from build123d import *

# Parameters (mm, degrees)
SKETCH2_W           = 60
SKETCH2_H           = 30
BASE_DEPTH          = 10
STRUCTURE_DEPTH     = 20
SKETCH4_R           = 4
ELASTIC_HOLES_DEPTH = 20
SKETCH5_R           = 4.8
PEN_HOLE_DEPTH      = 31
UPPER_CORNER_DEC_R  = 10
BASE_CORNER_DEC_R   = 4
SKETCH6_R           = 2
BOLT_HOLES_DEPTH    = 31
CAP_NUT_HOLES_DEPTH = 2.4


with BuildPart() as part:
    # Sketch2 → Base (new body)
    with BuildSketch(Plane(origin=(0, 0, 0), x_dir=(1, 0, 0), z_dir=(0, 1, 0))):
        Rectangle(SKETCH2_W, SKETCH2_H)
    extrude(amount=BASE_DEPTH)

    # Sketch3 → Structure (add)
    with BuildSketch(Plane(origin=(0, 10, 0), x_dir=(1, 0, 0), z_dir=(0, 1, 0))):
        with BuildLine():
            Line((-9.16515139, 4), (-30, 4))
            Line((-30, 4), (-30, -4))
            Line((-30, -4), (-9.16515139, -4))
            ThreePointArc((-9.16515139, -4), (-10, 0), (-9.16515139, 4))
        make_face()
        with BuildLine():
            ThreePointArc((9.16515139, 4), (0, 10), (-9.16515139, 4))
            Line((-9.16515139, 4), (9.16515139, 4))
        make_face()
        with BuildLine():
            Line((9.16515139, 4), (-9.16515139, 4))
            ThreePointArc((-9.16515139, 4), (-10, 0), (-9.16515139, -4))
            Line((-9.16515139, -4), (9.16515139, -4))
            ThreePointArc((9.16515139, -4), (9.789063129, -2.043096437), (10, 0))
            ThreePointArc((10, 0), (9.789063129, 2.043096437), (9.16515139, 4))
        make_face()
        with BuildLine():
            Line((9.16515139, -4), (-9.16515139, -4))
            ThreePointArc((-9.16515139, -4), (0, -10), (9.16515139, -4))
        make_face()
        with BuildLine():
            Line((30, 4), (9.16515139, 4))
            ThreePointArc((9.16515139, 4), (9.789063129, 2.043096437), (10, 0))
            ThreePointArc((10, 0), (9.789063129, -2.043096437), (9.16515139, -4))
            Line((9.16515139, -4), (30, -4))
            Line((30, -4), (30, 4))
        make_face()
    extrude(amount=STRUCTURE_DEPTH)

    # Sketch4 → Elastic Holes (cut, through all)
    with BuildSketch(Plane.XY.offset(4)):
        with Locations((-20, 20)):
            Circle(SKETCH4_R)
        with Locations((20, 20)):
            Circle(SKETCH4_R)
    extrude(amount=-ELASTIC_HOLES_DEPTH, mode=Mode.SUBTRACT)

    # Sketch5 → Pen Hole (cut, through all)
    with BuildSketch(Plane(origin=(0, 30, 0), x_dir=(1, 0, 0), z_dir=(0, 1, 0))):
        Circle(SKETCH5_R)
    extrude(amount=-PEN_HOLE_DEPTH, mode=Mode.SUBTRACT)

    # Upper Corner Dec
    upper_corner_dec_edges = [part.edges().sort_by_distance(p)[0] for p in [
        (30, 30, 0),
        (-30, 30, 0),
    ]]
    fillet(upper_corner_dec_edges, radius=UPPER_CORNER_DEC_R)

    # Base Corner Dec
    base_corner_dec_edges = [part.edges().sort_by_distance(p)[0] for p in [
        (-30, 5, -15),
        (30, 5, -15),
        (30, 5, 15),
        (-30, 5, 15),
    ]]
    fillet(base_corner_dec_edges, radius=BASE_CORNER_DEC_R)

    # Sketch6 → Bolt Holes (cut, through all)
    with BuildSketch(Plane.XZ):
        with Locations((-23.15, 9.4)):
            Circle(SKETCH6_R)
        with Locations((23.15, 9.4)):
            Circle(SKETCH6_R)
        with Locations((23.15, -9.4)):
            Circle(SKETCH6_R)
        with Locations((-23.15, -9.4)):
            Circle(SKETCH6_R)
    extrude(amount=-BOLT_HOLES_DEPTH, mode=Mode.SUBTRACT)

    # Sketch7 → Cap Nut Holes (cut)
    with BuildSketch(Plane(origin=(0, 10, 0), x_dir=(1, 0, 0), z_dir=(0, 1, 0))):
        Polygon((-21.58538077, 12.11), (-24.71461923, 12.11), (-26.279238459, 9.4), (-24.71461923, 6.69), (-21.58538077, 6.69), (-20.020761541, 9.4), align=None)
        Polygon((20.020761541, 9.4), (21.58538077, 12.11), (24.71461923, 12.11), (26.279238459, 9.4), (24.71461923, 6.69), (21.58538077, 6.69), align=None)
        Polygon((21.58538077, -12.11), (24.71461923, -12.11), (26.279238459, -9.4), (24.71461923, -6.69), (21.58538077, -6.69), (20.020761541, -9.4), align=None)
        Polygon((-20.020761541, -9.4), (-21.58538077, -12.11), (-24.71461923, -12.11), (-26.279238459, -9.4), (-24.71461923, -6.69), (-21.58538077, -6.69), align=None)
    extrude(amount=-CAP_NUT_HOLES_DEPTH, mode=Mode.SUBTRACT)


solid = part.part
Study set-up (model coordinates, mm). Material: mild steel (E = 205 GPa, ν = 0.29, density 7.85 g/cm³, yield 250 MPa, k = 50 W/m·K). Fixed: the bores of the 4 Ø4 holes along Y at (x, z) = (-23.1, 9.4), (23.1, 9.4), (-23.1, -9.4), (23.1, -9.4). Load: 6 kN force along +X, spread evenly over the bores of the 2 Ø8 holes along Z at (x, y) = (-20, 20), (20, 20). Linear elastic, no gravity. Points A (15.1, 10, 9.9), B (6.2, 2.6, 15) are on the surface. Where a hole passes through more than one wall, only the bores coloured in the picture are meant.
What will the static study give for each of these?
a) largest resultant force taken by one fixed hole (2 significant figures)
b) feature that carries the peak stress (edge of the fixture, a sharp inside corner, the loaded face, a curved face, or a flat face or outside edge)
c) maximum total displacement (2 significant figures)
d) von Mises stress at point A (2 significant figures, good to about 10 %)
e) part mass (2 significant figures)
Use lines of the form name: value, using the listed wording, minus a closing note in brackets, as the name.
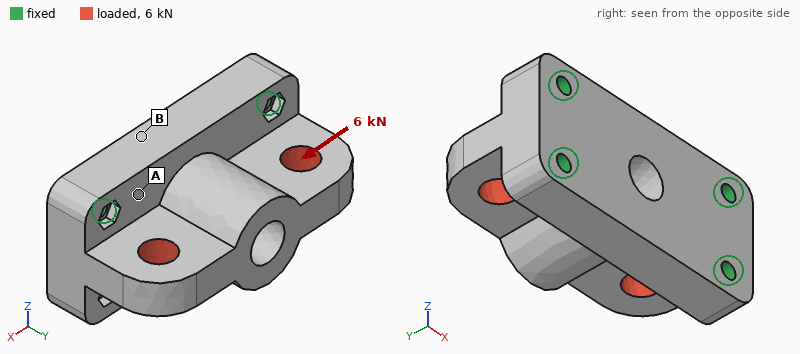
largest resultant force taken by one fixed hole: 1.8 kN
feature that carries the peak stress: edge of the fixture
maximum total displacement: 5.3 µm
von Mises stress at point A: 10 MPa
part mass: 210 g
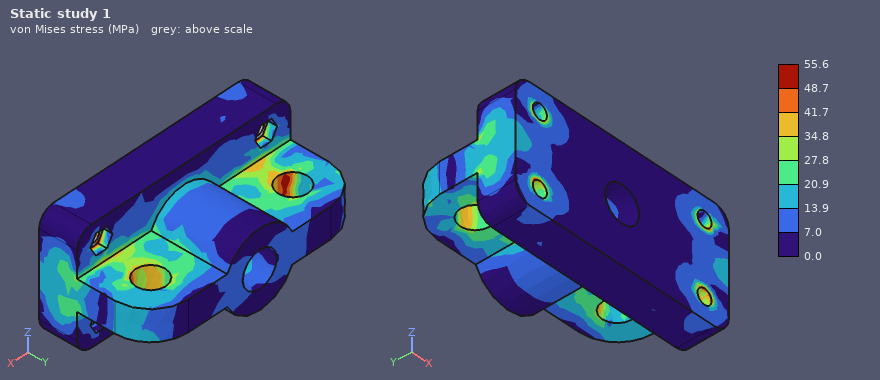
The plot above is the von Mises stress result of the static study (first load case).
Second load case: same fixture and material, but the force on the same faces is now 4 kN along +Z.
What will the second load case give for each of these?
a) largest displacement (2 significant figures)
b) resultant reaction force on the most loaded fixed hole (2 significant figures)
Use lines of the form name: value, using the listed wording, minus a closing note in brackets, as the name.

largest displacement: 13 µm
resultant reaction force on the most loaded fixed hole: 1.9 kN
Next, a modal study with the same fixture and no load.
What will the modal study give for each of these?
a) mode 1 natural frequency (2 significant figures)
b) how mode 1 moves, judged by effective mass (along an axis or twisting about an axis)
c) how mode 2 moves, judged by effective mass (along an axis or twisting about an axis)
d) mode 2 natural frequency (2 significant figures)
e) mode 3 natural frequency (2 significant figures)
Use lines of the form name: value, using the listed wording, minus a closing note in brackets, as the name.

mode 1 natural frequency: 11 kHz
how mode 1 moves, judged by effective mass: along Z
how mode 2 moves, judged by effective mass: along Y
mode 2 natural frequency: 17 kHz
mode 3 natural frequency: 20 kHz
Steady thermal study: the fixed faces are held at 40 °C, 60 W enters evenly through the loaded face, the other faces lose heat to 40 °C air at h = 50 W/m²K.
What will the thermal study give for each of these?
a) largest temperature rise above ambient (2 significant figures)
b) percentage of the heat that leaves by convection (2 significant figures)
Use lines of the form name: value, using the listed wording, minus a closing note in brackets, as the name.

largest temperature rise above ambient: 57 K
percentage of the heat that leaves by convection: 14 %
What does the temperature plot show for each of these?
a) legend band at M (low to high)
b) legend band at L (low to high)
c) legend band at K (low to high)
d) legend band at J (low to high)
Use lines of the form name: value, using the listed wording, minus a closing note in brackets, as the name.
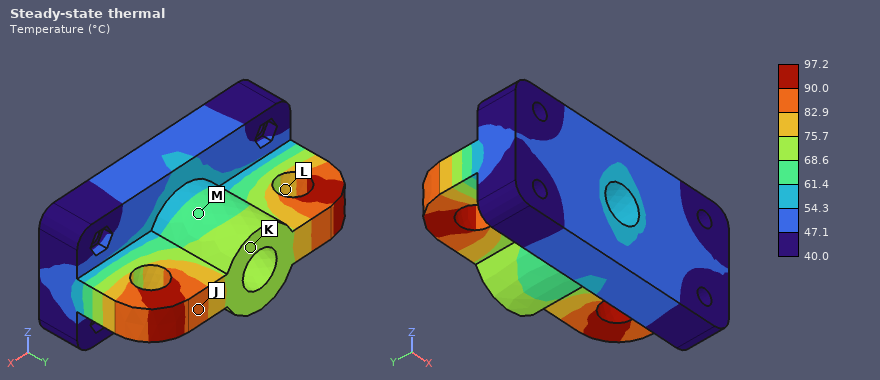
legend band at M: 61.4 to 68.6 °C
legend band at L: 75.7 to 82.9 °C
legend band at K: 68.6 to 75.7 °C
legend band at J: 82.9 to 90.0 °C
